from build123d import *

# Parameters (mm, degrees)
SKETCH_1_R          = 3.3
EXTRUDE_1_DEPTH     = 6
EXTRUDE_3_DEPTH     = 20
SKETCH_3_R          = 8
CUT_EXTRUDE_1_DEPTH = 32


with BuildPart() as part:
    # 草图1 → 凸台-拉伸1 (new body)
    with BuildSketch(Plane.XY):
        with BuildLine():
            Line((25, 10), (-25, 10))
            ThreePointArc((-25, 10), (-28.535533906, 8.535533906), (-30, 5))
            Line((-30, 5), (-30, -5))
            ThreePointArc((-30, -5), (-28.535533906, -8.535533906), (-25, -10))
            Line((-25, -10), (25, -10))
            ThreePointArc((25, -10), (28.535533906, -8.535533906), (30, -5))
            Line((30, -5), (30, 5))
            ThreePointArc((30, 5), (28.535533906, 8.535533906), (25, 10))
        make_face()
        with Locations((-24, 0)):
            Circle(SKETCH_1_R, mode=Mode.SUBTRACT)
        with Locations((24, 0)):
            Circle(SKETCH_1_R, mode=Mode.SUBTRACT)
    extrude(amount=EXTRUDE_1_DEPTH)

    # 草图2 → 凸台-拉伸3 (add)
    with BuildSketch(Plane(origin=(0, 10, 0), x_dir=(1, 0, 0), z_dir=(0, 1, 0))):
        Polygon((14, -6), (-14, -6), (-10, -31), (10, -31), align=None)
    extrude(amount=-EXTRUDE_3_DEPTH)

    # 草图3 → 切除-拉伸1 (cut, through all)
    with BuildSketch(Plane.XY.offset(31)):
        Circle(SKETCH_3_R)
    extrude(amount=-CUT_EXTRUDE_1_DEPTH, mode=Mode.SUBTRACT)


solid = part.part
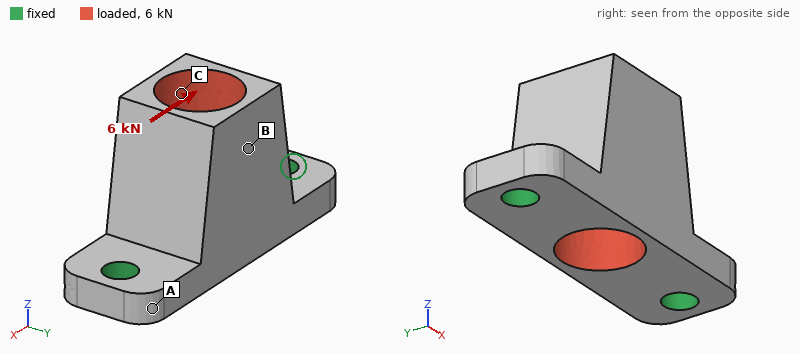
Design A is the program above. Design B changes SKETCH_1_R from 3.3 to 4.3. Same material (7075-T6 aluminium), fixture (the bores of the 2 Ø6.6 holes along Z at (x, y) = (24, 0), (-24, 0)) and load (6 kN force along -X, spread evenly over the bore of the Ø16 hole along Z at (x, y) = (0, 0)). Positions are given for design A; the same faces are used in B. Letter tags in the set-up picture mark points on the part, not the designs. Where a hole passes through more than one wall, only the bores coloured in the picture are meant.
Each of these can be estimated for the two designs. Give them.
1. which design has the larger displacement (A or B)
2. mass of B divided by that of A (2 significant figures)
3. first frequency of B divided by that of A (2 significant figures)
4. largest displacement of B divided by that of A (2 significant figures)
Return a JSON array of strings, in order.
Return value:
["A", "0.98", "1.1", "0.89"]
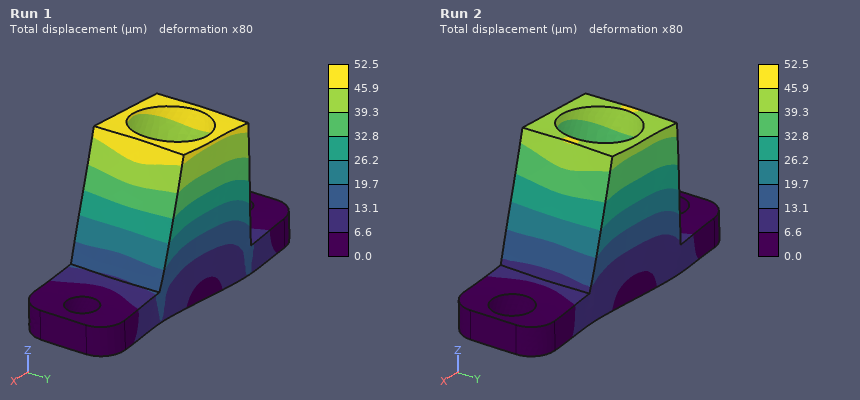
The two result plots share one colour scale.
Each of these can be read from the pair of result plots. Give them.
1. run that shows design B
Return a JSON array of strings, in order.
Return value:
["Run 2"]
